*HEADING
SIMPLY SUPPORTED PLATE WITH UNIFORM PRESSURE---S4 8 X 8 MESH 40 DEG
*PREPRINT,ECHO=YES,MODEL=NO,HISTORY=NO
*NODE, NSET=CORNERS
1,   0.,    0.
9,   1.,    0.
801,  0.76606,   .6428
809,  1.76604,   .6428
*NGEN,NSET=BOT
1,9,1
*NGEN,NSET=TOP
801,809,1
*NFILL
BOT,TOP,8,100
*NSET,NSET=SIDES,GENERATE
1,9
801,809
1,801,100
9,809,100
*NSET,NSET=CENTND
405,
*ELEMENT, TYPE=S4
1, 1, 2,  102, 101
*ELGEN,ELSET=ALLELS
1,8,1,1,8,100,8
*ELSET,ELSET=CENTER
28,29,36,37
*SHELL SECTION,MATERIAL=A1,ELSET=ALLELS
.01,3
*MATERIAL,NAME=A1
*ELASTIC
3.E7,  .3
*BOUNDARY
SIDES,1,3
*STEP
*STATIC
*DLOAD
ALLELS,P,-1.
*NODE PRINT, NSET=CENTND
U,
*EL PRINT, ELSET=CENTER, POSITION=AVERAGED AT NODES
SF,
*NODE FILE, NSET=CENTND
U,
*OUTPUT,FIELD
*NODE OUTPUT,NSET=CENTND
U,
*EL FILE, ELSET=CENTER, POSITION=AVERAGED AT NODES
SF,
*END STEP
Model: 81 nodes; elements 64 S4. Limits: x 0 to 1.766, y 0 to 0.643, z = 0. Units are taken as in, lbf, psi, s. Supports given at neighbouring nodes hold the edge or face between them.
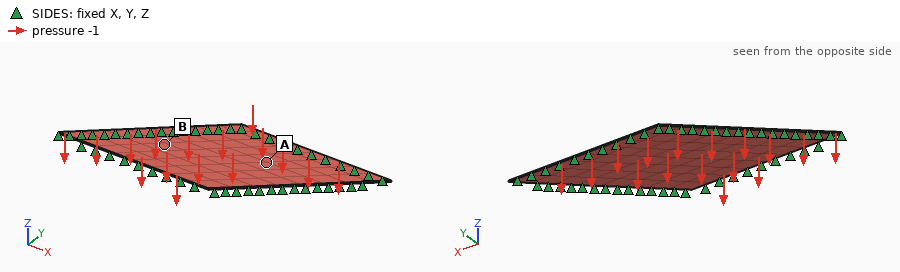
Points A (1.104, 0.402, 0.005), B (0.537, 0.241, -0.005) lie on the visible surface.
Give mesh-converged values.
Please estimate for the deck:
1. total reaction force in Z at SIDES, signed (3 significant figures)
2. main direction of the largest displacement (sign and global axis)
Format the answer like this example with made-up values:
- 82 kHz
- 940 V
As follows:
- 0.643 lbf
- -Z
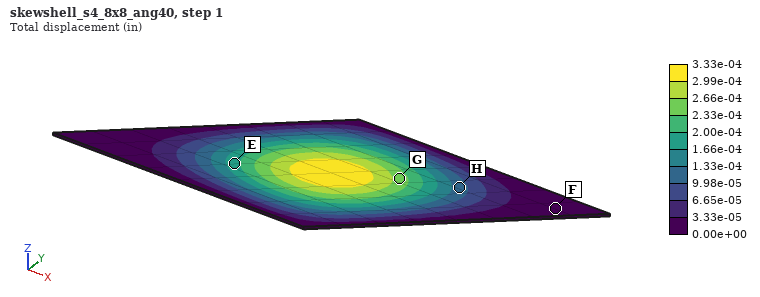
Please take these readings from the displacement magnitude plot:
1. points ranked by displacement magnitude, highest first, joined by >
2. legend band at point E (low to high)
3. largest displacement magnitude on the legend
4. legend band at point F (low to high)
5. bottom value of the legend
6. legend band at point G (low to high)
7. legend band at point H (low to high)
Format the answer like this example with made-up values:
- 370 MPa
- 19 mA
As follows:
- G > E > H > F
- 1.66e-04 to 2.00e-04 in
- 3.33e-04 in
- 0.00e+00 to 3.33e-05 in
- 0.00e+00 in
- 2.33e-04 to 2.66e-04 in
- 9.98e-05 to 1.33e-04 in
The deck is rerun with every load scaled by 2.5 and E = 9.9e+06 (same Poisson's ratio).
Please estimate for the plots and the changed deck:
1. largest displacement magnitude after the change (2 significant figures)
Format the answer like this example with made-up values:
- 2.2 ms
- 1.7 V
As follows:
- 0.0025 in
